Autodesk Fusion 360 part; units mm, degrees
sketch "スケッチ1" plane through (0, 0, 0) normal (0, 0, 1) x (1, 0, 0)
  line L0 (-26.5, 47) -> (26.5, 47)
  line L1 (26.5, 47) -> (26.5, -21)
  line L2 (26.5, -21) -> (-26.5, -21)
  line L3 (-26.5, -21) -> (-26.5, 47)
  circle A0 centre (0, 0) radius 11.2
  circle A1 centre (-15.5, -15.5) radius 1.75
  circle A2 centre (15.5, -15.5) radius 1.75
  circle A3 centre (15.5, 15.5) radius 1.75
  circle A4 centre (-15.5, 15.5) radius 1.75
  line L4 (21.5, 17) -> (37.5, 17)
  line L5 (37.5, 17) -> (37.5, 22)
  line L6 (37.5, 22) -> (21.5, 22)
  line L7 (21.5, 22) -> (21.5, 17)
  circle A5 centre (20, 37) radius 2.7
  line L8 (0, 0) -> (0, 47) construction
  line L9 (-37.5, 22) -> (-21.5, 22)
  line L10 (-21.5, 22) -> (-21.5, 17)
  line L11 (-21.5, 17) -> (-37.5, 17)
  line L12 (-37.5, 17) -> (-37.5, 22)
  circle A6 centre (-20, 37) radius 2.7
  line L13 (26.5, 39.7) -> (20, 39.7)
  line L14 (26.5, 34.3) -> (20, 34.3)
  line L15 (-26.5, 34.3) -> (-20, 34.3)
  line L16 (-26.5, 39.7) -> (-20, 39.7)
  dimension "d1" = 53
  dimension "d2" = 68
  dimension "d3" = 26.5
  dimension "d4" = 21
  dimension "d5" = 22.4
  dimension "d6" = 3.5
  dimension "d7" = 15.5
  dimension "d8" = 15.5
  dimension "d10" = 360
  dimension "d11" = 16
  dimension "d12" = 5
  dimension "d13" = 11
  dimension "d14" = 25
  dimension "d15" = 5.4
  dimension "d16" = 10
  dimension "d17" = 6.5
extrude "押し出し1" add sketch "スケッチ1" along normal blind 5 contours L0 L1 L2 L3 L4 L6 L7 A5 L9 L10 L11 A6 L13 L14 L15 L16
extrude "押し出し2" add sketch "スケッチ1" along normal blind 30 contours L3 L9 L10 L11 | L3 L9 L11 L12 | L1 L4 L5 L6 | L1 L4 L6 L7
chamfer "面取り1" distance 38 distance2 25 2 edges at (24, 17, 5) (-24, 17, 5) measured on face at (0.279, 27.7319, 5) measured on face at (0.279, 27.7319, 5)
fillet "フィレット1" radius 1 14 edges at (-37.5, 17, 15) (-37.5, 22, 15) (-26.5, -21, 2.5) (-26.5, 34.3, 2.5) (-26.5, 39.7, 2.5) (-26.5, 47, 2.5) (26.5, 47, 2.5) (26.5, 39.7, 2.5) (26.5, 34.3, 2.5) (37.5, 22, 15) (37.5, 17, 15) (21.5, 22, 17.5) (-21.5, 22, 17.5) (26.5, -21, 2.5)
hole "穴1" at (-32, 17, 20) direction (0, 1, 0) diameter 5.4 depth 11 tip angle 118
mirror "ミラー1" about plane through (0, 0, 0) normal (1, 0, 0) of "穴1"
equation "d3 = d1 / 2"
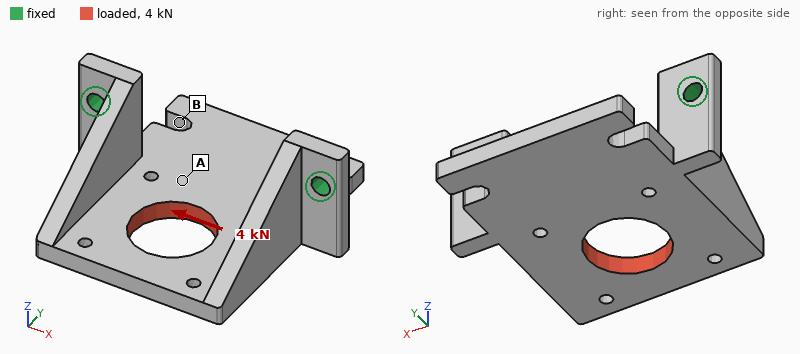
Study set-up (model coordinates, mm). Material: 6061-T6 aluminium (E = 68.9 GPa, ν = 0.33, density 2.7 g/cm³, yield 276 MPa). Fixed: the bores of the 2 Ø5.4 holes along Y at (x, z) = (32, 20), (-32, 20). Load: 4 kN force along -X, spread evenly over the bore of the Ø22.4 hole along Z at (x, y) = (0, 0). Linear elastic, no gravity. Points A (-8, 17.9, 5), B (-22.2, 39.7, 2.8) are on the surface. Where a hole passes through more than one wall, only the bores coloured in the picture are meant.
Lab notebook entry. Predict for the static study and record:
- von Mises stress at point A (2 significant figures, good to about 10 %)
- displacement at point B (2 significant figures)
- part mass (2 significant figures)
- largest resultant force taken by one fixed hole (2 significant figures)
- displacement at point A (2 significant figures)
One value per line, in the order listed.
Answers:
52 MPa
0.039 mm
66 g
2.4 kN
0.059 mm
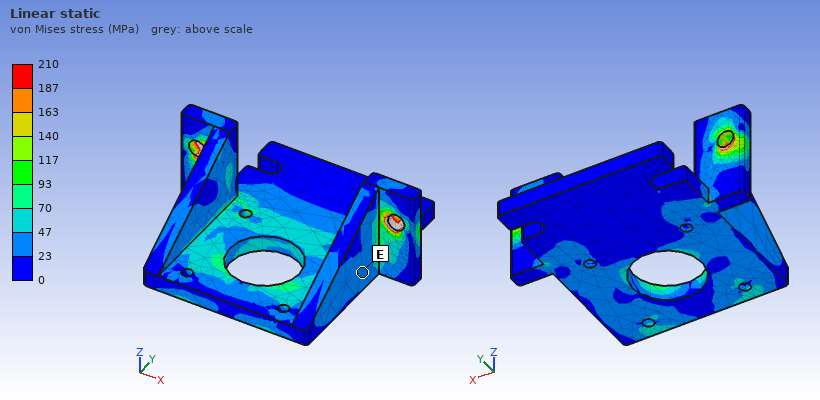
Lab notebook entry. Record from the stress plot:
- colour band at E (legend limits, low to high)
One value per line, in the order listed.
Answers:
23 to 47 MPa
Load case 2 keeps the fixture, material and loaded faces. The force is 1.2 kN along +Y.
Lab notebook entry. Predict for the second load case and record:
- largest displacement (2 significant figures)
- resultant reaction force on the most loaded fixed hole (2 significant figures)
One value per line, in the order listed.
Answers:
0.12 mm
610 N
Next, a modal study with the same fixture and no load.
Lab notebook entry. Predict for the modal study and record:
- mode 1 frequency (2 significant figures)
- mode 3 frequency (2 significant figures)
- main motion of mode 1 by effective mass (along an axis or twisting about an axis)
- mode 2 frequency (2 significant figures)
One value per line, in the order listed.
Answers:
2200 Hz
3800 Hz
along Y
3800 Hz
